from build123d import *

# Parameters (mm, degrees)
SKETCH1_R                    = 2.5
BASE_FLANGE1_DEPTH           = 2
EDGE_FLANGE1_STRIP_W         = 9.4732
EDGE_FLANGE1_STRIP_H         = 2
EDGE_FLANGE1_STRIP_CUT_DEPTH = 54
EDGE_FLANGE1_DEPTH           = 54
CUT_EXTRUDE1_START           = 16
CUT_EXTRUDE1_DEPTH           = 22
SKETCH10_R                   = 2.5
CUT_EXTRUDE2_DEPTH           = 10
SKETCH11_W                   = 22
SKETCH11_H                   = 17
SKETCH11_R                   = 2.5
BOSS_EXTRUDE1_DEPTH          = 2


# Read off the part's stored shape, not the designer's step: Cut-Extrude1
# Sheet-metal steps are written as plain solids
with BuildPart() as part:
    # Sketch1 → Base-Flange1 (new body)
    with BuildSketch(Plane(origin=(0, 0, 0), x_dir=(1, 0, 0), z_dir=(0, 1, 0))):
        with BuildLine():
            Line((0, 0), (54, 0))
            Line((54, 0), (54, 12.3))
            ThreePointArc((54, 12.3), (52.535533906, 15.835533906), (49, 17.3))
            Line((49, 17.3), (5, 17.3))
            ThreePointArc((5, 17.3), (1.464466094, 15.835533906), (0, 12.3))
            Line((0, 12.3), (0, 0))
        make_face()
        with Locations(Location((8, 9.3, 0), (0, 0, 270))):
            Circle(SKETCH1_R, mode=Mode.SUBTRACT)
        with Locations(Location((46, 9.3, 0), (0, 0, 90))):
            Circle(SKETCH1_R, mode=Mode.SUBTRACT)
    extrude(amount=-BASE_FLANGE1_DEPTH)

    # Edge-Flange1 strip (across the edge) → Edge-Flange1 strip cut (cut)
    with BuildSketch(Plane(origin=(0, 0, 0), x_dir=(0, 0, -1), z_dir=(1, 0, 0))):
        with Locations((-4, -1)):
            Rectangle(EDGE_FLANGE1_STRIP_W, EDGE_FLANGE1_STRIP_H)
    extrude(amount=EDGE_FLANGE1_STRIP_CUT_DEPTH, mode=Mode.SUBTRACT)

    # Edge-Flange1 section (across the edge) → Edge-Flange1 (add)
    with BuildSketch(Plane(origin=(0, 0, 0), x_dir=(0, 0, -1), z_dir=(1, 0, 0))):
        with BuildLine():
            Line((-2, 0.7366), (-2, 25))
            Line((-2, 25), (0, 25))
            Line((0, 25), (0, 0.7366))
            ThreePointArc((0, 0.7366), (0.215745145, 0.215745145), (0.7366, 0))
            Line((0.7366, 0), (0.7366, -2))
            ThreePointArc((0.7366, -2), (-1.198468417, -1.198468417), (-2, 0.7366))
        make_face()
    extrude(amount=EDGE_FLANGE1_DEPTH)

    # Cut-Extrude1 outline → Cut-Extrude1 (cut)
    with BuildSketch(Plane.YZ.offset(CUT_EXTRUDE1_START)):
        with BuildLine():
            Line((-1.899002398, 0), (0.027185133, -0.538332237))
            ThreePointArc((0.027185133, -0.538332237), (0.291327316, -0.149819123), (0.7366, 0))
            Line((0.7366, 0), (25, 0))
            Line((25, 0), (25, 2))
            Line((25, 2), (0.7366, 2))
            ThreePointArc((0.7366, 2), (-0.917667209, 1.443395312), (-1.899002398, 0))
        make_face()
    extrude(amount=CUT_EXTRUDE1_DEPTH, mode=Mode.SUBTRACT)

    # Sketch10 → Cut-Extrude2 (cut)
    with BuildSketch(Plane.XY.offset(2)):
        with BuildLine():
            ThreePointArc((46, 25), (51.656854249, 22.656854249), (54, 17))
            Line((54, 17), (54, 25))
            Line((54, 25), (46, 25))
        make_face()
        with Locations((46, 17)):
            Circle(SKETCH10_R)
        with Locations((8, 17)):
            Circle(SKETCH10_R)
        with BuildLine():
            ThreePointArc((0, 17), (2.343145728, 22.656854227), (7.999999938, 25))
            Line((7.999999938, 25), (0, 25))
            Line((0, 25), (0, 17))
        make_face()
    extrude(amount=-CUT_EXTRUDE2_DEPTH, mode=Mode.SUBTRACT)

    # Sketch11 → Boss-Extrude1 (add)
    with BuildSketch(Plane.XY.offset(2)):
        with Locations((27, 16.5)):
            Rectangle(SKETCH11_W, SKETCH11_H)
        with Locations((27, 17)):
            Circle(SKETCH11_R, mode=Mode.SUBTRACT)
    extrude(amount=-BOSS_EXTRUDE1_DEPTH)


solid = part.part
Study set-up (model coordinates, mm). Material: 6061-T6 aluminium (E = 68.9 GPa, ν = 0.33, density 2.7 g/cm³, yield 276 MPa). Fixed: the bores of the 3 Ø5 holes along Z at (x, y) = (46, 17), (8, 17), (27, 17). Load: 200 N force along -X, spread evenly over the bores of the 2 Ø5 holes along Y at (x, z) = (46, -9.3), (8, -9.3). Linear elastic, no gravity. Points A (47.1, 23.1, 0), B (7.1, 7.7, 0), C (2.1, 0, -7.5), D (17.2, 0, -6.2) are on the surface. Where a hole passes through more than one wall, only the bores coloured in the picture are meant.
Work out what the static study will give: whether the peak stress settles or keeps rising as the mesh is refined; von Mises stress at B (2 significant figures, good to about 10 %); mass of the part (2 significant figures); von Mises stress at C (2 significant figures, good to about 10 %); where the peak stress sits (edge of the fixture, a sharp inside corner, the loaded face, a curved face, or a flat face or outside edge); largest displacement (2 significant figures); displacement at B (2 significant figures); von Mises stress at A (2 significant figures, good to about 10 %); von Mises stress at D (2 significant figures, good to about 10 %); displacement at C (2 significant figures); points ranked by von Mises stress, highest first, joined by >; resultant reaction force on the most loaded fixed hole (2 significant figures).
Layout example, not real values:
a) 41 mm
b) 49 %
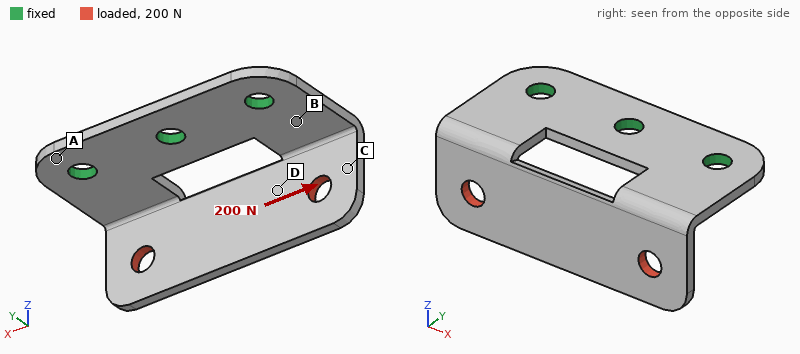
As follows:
a) keeps rising
b) 24 MPa
c) 11 g
d) 13 MPa
e) a sharp inside corner
f) 0.10 mm
g) 0.018 mm
h) 5.6 MPa
i) 17 MPa
j) 0.076 mm
k) B > D > C > A
l) 100 N
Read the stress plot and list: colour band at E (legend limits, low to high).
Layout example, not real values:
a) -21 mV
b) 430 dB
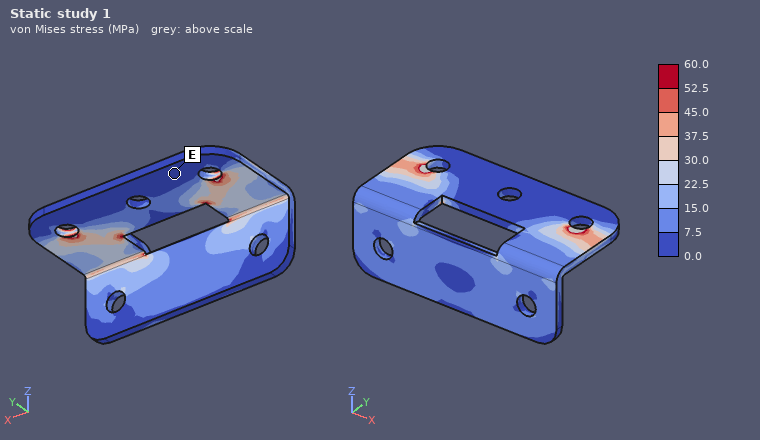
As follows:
a) 0.0 to 7.5 MPa
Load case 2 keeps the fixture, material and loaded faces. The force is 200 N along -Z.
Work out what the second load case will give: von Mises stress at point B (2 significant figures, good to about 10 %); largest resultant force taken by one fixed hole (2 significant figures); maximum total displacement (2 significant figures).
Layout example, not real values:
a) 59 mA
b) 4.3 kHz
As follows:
a) 65 MPa
b) 94 N
c) 0.34 mm
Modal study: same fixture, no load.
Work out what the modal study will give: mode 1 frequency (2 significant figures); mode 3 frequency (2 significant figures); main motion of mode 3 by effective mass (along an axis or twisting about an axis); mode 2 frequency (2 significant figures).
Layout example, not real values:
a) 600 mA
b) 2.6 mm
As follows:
a) 1600 Hz
b) 4200 Hz
c) along Z
d) 2800 Hz
